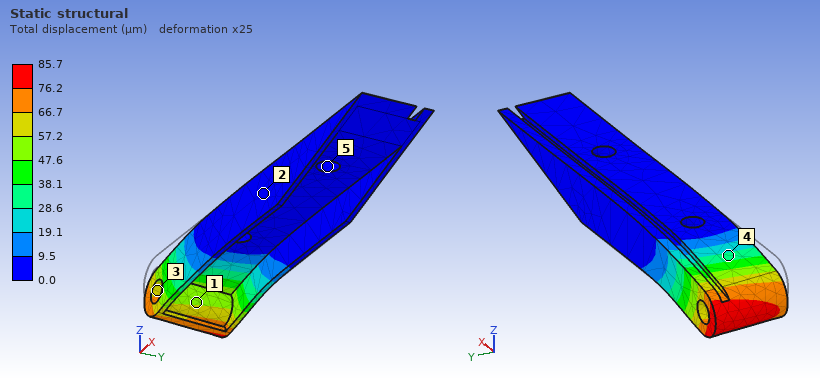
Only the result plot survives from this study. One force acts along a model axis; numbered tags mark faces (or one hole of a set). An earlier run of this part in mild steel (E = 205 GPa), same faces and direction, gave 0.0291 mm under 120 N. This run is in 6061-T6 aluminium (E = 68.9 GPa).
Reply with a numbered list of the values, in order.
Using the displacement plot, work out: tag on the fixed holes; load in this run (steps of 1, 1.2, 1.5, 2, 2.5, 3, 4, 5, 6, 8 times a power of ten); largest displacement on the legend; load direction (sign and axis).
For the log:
1. 5
2. 120 N
3. 85.7 µm
4. -Z
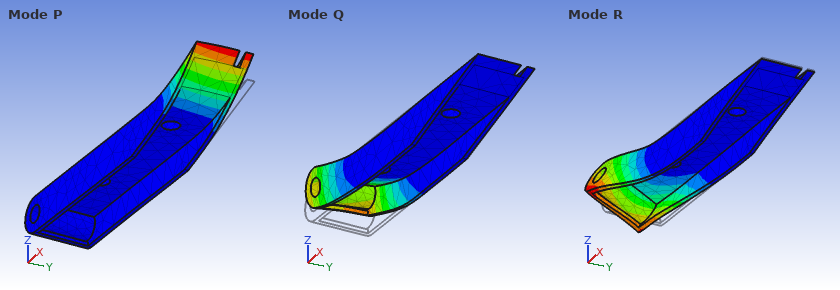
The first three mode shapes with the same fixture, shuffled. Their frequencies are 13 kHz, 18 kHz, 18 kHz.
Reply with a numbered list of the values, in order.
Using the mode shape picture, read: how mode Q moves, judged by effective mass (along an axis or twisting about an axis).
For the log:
1. along Z
